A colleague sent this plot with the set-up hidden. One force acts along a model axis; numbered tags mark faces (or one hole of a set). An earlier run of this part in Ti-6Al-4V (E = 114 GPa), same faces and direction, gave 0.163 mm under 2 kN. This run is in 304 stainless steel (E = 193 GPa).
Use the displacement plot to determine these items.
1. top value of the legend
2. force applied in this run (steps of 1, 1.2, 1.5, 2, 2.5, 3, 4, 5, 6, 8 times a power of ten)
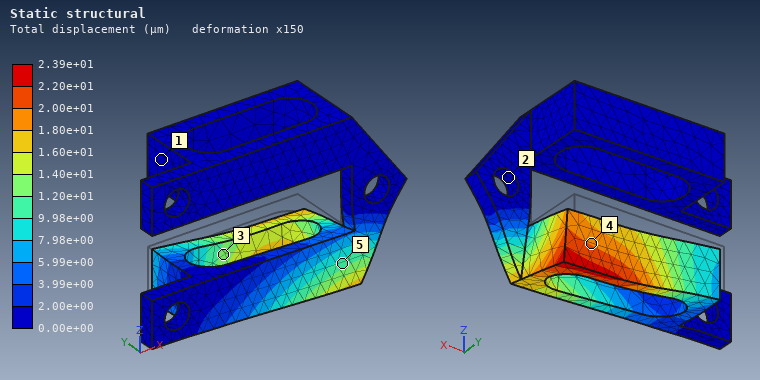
2.39e+01 µm
500 N
